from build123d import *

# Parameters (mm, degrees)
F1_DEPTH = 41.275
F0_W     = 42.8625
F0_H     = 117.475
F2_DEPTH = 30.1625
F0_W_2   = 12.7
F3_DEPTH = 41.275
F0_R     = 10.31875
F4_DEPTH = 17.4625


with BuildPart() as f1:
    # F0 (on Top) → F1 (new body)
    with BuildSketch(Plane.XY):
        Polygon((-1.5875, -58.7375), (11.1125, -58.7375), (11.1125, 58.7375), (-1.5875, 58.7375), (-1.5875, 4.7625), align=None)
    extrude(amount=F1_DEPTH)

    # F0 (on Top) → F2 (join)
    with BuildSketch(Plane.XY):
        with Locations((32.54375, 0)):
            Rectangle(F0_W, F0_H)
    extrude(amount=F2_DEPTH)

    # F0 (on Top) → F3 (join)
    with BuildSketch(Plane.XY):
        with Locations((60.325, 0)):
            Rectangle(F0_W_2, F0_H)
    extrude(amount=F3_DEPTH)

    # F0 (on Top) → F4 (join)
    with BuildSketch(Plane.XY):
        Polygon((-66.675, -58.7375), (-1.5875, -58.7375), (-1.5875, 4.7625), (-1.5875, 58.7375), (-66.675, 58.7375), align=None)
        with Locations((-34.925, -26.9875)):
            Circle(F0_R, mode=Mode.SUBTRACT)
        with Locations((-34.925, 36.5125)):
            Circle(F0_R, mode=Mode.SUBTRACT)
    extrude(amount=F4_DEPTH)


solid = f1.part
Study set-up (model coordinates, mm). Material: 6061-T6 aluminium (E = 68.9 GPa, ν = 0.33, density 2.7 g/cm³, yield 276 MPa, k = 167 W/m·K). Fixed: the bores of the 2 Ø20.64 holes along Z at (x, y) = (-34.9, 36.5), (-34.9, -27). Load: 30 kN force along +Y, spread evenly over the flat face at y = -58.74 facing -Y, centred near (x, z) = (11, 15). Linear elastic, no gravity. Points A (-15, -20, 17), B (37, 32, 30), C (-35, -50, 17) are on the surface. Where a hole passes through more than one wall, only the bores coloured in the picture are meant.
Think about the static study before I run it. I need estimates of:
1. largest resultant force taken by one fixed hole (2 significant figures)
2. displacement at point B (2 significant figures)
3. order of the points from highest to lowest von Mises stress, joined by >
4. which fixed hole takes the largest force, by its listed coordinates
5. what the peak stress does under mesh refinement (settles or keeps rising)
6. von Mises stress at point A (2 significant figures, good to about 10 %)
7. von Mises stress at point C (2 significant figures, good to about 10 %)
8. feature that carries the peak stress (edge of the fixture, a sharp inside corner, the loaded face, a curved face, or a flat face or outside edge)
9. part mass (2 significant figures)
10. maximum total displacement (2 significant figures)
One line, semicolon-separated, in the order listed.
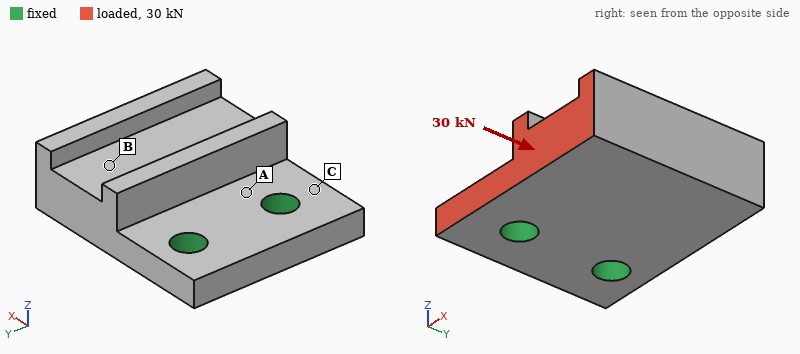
26 kN; 44 µm; A > C > B; (-34.9, -27); keeps rising; 37 MPa; 19 MPa; edge of the fixture; 1.1 kg; 72 µm
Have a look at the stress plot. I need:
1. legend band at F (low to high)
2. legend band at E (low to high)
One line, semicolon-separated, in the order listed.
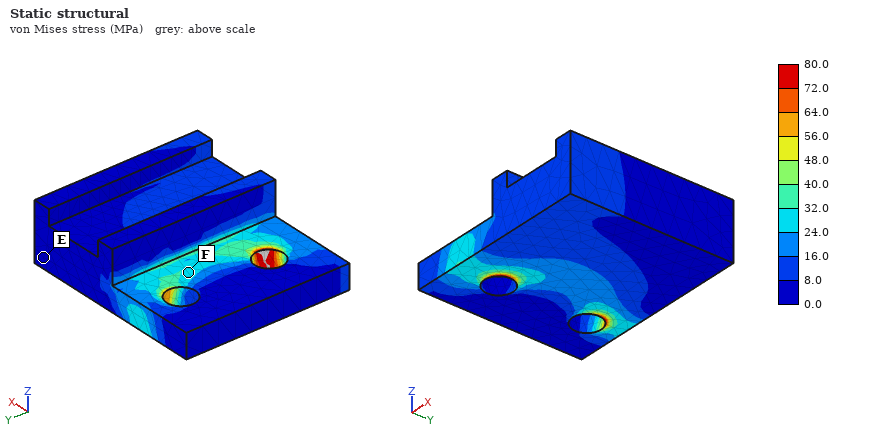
24.0 to 32.0 MPa; 0.0 to 8.0 MPa
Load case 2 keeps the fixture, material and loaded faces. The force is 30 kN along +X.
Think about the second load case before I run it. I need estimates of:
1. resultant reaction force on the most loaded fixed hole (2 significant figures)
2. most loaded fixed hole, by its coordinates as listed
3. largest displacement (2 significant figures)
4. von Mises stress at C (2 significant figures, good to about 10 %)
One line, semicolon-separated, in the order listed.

40 kN; (-34.9, -27); 0.22 mm; 37 MPa
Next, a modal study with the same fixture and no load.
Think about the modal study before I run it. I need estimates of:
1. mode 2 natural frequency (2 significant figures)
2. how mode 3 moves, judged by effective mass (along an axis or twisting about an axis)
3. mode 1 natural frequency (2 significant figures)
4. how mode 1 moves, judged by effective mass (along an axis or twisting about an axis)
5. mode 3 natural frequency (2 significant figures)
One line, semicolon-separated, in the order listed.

3000 Hz; along Y; 1100 Hz; along Z; 4000 Hz
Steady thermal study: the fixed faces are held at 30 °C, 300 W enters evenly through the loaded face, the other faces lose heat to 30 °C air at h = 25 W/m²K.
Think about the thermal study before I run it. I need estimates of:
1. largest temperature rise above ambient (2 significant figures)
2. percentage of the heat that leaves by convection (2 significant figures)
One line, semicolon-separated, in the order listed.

51 K; 7.4 %
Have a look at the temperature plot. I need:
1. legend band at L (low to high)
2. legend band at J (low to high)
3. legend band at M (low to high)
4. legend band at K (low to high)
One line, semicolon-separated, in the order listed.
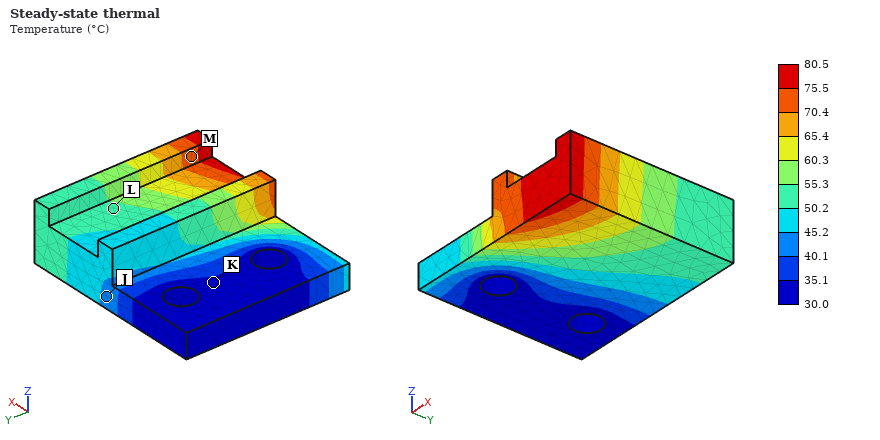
50.2 to 55.3 °C; 40.1 to 45.2 °C; 70.4 to 75.5 °C; 30.0 to 35.1 °C
